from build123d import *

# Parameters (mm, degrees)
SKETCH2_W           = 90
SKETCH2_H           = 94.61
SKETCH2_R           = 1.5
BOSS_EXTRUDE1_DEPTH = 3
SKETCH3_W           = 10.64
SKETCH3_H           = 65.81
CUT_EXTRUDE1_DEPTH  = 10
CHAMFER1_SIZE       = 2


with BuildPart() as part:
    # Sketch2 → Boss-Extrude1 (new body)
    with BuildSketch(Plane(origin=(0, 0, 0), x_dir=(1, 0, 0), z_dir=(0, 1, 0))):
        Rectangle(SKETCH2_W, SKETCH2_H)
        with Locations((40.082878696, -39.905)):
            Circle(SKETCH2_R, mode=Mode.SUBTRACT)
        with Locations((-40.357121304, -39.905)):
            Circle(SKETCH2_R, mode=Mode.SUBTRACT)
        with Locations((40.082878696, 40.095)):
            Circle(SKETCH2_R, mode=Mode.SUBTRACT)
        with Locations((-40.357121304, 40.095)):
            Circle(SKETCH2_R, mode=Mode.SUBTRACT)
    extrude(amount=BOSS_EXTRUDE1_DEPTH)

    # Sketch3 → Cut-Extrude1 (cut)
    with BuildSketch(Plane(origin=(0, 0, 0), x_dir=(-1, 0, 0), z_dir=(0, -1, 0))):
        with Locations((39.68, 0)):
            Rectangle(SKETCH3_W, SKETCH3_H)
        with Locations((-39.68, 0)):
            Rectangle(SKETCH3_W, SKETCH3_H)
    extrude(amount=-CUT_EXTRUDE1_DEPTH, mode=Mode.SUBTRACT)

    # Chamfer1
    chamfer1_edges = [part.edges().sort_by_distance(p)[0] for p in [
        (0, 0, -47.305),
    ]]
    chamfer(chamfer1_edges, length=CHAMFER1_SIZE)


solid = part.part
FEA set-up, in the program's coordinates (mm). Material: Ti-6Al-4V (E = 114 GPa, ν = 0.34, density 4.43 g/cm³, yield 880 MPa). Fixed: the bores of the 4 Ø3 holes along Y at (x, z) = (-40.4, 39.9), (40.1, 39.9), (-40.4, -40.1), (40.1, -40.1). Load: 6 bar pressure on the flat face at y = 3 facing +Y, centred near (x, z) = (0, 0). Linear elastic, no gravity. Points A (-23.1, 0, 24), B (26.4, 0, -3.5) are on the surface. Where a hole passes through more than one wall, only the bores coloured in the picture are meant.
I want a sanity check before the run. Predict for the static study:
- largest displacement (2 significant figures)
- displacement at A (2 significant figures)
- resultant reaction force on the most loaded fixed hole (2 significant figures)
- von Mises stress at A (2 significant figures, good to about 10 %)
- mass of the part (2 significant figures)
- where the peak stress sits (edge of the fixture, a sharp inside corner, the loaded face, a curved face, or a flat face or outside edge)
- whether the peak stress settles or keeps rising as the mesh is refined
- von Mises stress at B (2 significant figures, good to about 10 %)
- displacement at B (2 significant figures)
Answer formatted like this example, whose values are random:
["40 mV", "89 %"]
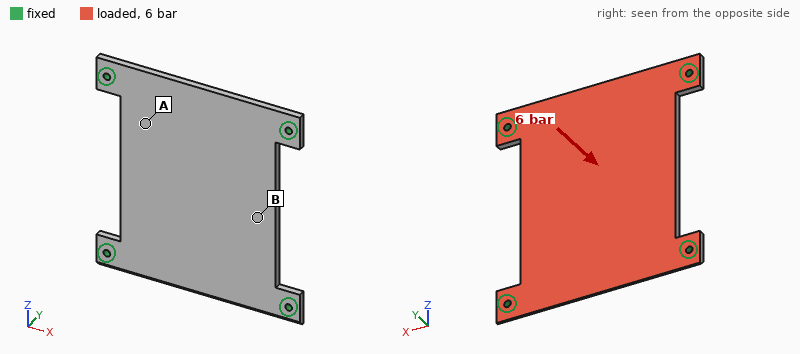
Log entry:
["0.82 mm", "0.47 mm", "1.1 kN", "98 MPa", "93 g", "edge of the fixture", "keeps rising", "160 MPa", "0.66 mm"]
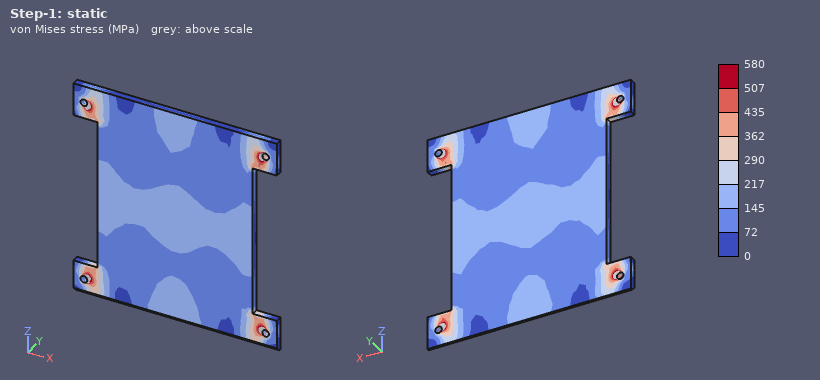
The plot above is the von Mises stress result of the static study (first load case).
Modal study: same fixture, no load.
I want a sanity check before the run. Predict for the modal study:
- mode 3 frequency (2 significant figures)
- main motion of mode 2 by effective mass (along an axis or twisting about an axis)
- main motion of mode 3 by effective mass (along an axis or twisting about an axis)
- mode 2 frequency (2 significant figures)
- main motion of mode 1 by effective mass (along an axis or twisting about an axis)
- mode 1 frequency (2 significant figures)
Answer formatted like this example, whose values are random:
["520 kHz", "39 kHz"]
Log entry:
["2700 Hz", "twisting about X", "twisting about Z", "2500 Hz", "along Y", "1400 Hz"]
